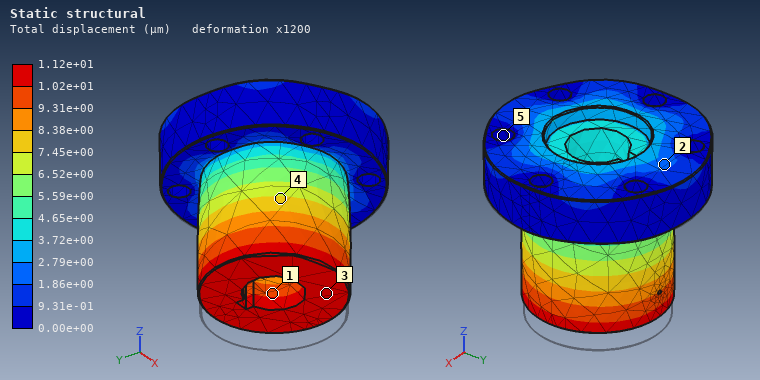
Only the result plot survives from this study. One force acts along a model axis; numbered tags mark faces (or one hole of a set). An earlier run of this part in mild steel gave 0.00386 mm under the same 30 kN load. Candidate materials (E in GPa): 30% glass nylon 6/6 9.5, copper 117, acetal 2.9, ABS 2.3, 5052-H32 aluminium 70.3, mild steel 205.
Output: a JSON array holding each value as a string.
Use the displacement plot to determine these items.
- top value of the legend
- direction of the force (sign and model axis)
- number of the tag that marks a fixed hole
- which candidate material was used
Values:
["1.12e+01 µm", "+Z", "5", "5052-H32 aluminium"]
